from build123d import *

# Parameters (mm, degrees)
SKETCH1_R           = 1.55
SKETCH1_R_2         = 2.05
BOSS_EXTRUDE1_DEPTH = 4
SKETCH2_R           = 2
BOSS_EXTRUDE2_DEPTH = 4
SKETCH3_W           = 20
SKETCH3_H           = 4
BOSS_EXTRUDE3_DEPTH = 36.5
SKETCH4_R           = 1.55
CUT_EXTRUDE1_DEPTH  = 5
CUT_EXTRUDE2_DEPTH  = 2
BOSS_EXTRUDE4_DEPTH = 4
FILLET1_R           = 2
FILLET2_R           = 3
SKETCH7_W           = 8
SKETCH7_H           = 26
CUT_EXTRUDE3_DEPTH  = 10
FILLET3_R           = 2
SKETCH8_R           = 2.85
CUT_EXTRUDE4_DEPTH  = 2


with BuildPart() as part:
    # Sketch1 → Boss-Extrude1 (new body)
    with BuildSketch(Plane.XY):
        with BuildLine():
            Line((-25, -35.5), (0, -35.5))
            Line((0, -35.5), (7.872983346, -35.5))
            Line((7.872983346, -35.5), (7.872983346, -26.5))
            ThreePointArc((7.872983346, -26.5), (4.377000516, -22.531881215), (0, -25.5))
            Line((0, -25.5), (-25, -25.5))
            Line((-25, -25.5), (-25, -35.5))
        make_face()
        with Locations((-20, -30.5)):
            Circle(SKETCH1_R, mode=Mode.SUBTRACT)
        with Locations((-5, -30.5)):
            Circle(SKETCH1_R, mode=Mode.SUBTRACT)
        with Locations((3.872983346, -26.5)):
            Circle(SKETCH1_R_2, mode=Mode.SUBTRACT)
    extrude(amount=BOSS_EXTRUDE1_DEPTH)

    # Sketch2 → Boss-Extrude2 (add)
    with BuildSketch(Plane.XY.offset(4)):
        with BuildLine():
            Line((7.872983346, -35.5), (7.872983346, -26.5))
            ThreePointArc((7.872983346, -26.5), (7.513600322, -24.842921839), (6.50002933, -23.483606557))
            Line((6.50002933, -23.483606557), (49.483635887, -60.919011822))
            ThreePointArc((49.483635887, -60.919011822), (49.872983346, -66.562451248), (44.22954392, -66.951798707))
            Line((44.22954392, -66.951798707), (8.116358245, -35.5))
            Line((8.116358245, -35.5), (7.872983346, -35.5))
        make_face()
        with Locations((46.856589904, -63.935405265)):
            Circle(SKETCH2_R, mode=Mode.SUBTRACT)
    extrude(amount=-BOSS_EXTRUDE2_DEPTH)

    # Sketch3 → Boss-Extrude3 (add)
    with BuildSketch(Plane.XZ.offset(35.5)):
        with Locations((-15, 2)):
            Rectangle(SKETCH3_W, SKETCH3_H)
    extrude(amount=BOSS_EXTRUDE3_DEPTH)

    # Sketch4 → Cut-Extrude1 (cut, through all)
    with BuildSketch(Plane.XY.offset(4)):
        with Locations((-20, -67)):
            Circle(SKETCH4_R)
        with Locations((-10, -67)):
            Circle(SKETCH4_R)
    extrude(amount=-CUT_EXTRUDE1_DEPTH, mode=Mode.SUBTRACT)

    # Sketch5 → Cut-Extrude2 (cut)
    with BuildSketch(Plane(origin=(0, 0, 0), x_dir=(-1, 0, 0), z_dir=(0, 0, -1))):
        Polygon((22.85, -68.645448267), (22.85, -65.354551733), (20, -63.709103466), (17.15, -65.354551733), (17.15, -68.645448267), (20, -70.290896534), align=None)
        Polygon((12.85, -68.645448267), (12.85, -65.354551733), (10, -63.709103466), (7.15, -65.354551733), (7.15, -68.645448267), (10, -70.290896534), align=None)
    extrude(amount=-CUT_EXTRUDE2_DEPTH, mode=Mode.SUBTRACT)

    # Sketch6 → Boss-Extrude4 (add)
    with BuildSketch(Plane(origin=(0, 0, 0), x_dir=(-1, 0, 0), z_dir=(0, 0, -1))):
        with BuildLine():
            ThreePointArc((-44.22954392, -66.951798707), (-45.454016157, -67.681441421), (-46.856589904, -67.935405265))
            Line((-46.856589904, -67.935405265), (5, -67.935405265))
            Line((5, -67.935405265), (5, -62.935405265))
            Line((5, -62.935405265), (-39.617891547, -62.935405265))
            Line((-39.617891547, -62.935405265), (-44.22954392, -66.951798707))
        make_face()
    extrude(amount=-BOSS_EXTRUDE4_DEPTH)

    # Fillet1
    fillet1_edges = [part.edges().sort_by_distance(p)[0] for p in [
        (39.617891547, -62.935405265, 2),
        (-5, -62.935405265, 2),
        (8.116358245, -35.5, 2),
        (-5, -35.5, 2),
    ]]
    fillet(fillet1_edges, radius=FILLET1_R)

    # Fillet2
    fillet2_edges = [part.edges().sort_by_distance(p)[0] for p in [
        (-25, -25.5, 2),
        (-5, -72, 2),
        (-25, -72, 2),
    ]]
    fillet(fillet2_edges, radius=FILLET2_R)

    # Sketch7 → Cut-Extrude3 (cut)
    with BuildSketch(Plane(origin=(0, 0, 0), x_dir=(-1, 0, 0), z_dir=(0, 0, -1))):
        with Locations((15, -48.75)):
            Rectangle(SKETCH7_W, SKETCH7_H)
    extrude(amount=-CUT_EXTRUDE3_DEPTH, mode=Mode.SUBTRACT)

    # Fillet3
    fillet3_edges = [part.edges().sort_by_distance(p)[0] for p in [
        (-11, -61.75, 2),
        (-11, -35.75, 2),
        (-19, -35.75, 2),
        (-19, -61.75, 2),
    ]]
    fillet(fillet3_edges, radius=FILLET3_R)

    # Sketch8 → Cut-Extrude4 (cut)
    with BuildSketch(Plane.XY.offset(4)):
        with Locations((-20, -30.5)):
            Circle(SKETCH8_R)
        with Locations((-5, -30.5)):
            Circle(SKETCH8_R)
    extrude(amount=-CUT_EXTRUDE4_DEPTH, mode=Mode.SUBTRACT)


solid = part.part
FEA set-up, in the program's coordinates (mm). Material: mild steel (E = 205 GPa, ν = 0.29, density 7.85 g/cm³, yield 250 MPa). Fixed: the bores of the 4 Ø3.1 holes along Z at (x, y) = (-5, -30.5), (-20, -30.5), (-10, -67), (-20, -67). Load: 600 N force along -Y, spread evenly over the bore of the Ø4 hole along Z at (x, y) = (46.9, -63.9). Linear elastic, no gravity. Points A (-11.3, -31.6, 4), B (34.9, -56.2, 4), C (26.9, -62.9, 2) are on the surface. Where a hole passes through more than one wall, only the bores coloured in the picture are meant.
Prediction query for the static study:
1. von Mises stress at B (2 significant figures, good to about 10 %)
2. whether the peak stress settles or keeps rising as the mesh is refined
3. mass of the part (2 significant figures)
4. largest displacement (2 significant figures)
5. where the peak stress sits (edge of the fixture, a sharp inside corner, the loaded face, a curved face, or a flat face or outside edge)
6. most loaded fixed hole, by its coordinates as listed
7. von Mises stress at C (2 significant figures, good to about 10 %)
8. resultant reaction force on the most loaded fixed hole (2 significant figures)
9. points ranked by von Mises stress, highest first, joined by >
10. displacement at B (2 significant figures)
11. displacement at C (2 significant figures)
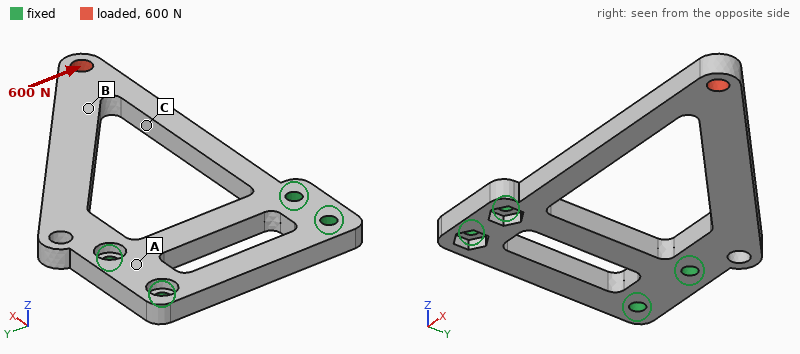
31 MPa
keeps rising
46 g
46 µm
edge of the fixture
(-5, -30.5)
58 MPa
980 N
C > B > A
37 µm
31 µm
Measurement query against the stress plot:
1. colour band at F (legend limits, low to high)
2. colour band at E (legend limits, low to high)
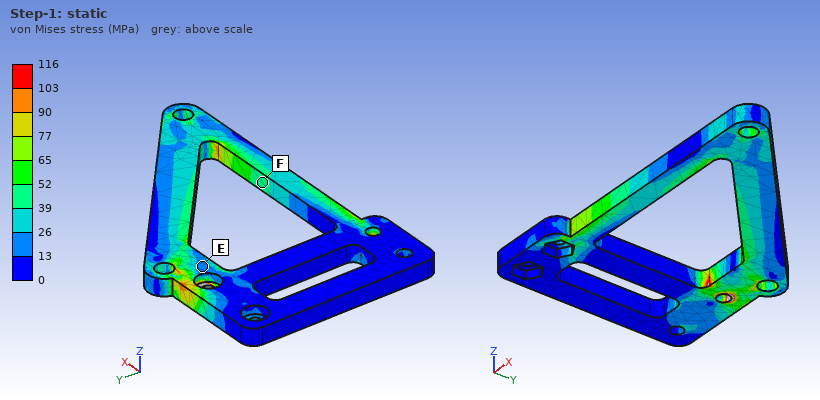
39 to 52 MPa
13 to 26 MPa
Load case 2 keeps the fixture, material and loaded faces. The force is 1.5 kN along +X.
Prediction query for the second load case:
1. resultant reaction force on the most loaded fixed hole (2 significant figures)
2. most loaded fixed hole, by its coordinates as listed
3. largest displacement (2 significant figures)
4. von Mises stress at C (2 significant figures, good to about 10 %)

1.1 kN
(-10, -67)
36 µm
83 MPa
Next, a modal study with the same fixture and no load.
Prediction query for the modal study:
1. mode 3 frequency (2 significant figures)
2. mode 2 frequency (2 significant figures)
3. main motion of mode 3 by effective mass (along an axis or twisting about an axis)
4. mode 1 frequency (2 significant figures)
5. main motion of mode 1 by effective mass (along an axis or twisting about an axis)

4900 Hz
4200 Hz
along Y
930 Hz
along Z
